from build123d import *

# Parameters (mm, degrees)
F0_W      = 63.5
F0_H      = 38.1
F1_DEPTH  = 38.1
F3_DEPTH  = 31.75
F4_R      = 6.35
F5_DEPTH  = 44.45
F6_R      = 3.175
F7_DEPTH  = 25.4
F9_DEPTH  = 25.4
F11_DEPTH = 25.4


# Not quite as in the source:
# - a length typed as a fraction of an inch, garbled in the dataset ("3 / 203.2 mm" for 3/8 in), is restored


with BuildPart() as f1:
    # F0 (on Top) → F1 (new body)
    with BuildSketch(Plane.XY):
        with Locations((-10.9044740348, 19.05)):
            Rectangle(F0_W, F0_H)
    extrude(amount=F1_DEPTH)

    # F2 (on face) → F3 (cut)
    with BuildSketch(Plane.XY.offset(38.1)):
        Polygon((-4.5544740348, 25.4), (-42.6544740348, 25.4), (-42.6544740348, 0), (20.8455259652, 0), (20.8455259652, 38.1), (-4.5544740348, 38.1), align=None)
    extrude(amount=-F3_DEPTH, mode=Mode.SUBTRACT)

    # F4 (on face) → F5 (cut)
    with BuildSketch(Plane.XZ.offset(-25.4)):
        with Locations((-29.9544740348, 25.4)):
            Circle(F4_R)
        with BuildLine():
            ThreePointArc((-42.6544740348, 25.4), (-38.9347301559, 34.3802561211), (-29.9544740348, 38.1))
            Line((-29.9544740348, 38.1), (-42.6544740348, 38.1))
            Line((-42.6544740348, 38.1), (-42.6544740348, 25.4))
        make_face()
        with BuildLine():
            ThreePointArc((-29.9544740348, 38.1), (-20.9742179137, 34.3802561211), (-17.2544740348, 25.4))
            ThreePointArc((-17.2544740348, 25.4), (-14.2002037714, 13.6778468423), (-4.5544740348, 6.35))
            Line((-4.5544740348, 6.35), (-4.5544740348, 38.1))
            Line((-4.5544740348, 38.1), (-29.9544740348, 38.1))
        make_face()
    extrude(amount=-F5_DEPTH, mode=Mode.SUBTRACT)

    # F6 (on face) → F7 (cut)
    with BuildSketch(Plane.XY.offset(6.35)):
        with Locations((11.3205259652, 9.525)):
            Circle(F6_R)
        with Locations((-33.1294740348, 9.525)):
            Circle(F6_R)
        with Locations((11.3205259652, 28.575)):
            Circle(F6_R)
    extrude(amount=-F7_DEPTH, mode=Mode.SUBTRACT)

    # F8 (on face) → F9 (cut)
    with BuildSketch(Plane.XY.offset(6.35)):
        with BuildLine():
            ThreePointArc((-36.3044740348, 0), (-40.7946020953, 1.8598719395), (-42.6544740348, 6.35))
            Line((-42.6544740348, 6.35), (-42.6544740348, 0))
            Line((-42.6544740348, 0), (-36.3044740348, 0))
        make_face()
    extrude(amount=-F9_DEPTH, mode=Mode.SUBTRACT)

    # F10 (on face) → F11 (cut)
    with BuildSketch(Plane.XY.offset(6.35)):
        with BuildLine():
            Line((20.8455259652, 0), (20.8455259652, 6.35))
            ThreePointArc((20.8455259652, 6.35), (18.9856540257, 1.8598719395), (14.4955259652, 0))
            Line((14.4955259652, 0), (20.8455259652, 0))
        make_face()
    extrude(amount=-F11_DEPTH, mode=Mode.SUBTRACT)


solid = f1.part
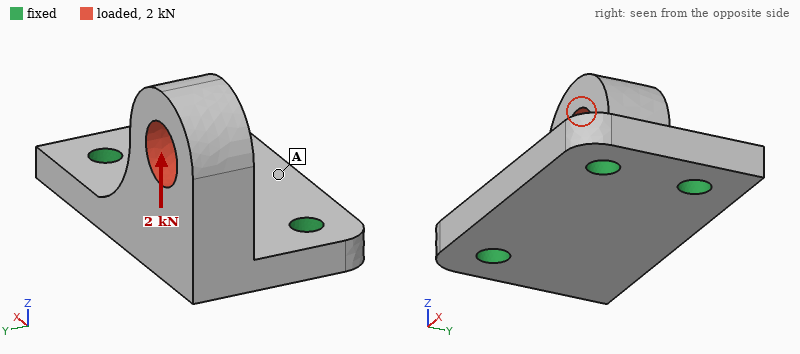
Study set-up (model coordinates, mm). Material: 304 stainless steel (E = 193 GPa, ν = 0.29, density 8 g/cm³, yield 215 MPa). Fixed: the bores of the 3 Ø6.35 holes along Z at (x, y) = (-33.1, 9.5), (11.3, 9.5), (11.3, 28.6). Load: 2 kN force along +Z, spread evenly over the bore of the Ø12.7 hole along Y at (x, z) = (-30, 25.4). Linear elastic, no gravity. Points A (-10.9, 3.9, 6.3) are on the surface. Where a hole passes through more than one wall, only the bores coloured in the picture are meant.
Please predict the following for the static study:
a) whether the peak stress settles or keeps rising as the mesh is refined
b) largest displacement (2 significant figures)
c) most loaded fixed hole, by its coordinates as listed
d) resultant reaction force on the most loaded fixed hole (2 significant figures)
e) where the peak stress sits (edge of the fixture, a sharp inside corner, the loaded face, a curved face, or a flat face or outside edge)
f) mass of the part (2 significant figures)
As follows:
keeps rising
76 µm
(-33.1, 9.5)
1.6 kN
edge of the fixture
190 g
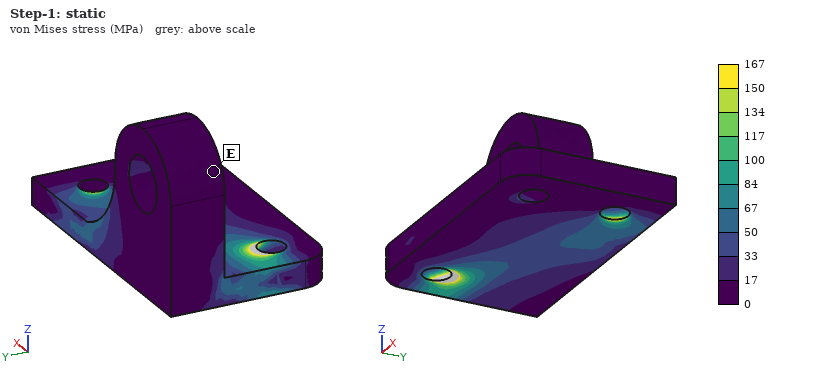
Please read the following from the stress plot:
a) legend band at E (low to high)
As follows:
0 to 17 MPa
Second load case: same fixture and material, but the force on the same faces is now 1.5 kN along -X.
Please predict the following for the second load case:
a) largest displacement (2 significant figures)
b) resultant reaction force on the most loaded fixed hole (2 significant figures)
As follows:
37 µm
960 N
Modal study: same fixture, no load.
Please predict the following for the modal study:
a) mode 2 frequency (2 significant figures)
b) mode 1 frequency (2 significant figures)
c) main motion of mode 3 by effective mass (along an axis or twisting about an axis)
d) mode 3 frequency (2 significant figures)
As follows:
6500 Hz
2900 Hz
along Z
8800 Hz
